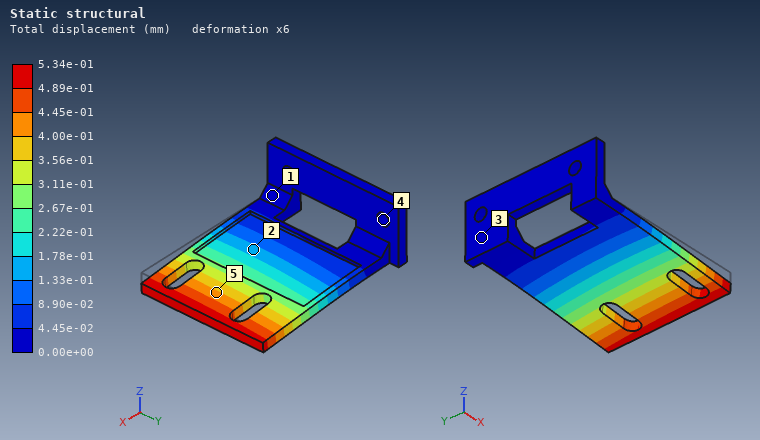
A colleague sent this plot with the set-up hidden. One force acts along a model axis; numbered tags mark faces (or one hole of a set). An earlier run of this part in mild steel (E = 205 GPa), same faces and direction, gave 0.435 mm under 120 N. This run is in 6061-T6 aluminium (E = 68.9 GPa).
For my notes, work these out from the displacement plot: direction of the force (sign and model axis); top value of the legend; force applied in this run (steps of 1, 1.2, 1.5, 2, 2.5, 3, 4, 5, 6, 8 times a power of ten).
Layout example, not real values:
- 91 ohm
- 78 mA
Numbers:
- -Z
- 5.34e-01 mm
- 50 N
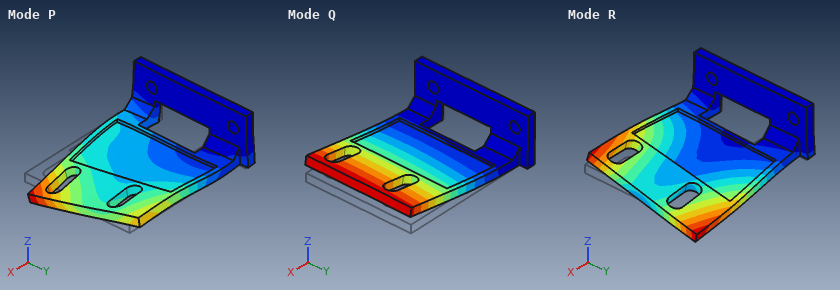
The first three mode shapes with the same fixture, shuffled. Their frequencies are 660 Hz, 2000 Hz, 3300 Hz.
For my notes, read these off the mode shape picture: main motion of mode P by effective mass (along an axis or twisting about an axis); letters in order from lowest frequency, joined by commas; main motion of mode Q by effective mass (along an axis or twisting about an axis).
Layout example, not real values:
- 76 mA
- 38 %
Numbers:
- along Y
- Q, R, P
- along Z
